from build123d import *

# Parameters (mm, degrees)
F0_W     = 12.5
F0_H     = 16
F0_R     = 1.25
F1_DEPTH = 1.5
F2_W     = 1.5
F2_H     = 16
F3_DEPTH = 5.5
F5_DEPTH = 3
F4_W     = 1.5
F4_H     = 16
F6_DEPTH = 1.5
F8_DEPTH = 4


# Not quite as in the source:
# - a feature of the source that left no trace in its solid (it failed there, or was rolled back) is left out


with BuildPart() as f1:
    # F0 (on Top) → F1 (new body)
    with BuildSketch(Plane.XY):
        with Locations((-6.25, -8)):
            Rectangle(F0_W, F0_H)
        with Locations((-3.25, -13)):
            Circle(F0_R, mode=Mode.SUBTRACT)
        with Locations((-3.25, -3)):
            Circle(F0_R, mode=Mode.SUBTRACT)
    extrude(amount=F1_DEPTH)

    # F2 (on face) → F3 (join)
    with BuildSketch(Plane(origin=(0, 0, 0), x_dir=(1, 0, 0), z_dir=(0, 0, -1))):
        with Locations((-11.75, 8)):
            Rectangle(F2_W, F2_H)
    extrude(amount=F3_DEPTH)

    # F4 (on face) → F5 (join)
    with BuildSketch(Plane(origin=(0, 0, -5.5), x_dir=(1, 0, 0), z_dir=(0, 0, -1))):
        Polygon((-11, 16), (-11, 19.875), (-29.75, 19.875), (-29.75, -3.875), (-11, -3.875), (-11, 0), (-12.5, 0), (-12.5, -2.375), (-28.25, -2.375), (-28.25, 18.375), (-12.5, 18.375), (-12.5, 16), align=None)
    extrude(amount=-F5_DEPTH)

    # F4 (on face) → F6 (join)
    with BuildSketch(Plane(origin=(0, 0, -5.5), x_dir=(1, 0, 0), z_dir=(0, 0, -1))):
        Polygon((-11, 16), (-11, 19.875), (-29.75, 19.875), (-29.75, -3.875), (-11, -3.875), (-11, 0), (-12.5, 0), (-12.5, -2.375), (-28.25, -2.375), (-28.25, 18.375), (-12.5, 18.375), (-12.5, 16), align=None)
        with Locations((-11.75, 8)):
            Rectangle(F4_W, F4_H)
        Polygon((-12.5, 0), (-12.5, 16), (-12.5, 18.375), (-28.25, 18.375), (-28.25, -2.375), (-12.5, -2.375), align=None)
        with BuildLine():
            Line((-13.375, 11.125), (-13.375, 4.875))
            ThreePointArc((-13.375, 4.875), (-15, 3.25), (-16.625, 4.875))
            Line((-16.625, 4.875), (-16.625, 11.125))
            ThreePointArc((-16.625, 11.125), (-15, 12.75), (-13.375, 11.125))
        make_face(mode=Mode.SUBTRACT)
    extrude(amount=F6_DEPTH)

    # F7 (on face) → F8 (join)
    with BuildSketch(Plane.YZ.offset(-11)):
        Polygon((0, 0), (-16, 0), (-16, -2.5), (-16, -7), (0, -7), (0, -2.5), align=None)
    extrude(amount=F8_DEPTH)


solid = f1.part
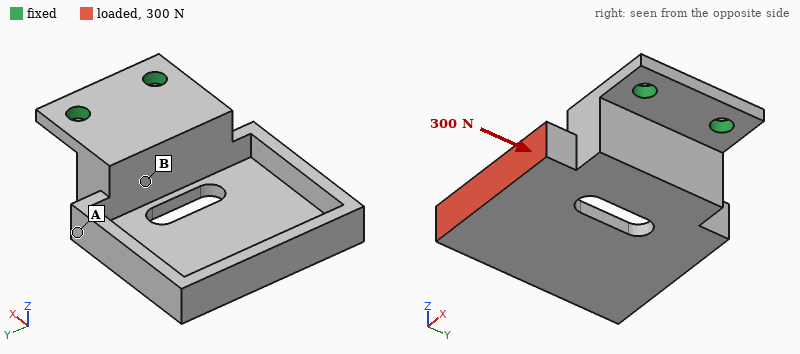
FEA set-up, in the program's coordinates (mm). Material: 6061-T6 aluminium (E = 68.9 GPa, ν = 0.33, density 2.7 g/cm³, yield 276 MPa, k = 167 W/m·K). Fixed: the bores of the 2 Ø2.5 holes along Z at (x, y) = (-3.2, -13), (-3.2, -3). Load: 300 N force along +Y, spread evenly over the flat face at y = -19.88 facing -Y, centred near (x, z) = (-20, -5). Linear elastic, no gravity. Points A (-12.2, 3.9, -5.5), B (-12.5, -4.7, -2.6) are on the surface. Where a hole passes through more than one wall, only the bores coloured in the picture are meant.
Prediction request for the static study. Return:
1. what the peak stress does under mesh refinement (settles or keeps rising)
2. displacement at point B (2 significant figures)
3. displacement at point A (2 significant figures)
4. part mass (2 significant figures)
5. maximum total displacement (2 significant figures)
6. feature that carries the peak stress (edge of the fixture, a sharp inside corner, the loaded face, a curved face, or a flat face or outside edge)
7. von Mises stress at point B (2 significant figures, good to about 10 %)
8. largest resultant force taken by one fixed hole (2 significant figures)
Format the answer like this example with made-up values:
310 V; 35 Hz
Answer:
keeps rising; 13 µm; 32 µm; 4.8 g; 85 µm; edge of the fixture; 40 MPa; 500 N
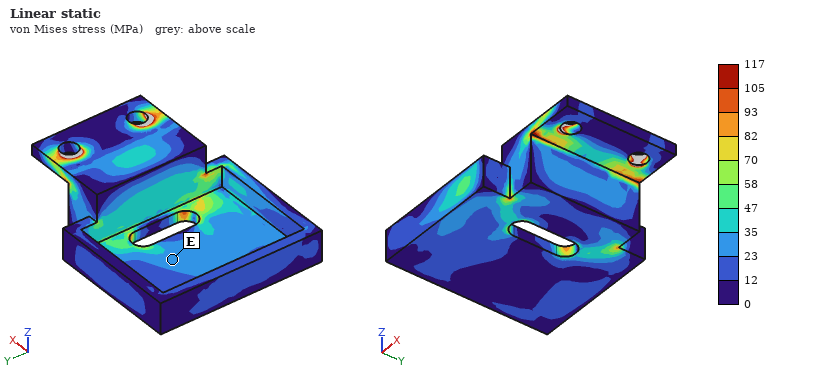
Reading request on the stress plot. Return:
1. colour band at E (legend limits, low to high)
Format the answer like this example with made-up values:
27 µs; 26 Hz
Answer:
23 to 35 MPa
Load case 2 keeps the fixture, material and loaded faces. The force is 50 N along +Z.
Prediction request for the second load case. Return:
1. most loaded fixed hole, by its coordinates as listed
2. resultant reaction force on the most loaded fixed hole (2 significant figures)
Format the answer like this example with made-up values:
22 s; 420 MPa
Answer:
(-3.2, -13); 79 N
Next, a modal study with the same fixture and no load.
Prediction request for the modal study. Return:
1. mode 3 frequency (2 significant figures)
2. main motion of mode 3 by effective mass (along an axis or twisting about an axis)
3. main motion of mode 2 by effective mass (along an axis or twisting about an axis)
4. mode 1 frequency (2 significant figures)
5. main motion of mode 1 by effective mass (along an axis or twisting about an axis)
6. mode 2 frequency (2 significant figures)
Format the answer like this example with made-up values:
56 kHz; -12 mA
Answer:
7200 Hz; along Y; twisting about X; 1500 Hz; along Z; 5600 Hz
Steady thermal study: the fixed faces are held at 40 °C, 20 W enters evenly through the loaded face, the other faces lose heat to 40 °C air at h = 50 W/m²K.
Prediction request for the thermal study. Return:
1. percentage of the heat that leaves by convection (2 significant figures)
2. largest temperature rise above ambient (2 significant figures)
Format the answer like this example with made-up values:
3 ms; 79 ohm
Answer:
18 %; 80 K
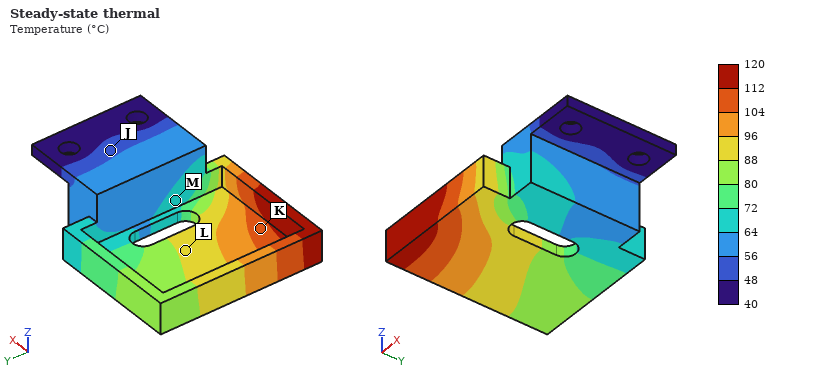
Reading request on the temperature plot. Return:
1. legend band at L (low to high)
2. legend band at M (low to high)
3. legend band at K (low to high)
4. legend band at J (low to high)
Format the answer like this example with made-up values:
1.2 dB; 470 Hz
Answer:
88 to 96 °C; 64 to 72 °C; 104 to 112 °C; 48 to 56 °C
